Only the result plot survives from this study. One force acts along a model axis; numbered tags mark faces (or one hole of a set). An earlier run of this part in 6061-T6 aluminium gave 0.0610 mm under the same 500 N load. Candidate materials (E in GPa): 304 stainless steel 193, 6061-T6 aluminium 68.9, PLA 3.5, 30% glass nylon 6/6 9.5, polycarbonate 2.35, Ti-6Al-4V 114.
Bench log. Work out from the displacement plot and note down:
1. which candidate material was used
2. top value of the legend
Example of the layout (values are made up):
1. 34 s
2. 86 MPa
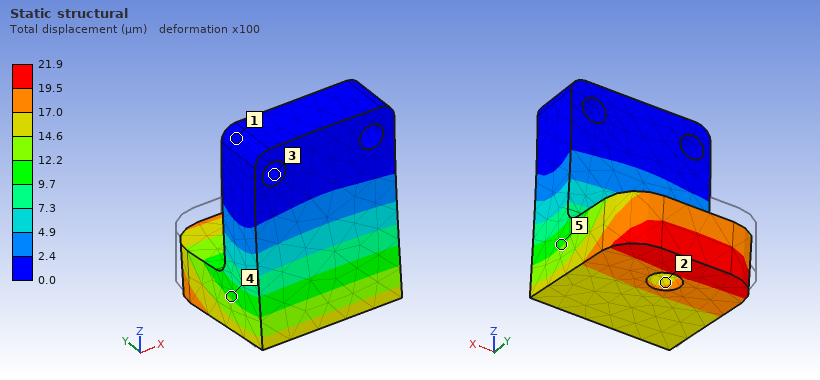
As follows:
1. 304 stainless steel
2. 21.9 µm
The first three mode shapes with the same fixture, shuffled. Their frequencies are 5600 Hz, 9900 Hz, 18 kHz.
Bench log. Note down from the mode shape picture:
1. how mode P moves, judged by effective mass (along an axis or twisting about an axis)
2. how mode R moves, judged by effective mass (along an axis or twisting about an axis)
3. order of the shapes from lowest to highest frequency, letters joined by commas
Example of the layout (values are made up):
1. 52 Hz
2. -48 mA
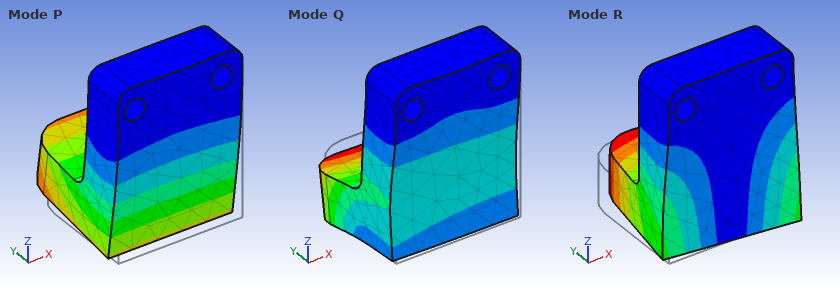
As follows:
1. along Y
2. along X
3. P, R, Q
